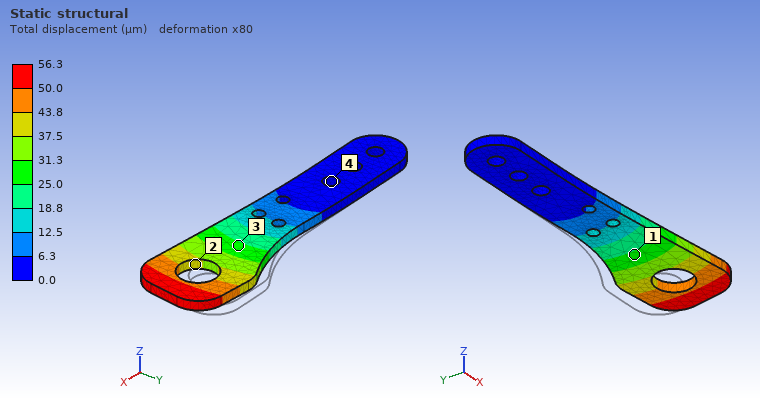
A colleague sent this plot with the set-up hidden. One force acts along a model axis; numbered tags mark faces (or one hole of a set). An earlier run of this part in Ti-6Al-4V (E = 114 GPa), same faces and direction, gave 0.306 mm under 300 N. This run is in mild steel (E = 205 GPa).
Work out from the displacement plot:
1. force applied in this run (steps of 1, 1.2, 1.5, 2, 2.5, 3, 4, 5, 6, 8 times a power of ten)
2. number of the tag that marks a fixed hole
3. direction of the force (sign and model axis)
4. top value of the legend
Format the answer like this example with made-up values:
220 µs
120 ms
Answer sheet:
100 N
4
-Y
56.3 µm
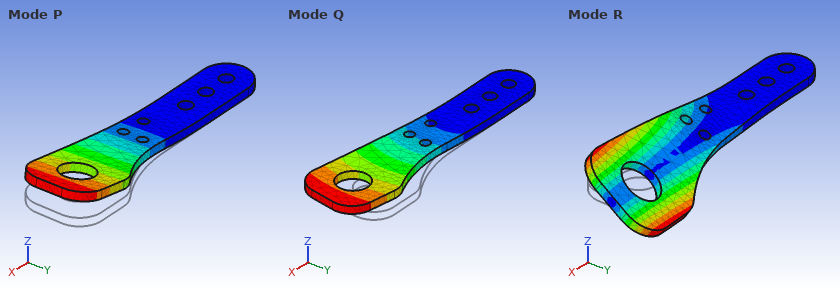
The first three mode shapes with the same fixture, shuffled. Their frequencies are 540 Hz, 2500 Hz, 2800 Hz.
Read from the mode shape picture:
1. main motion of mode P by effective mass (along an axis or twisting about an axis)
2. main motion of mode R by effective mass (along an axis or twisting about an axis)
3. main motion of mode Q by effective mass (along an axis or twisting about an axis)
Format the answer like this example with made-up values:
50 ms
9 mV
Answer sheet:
along Z
twisting about X
along Y
